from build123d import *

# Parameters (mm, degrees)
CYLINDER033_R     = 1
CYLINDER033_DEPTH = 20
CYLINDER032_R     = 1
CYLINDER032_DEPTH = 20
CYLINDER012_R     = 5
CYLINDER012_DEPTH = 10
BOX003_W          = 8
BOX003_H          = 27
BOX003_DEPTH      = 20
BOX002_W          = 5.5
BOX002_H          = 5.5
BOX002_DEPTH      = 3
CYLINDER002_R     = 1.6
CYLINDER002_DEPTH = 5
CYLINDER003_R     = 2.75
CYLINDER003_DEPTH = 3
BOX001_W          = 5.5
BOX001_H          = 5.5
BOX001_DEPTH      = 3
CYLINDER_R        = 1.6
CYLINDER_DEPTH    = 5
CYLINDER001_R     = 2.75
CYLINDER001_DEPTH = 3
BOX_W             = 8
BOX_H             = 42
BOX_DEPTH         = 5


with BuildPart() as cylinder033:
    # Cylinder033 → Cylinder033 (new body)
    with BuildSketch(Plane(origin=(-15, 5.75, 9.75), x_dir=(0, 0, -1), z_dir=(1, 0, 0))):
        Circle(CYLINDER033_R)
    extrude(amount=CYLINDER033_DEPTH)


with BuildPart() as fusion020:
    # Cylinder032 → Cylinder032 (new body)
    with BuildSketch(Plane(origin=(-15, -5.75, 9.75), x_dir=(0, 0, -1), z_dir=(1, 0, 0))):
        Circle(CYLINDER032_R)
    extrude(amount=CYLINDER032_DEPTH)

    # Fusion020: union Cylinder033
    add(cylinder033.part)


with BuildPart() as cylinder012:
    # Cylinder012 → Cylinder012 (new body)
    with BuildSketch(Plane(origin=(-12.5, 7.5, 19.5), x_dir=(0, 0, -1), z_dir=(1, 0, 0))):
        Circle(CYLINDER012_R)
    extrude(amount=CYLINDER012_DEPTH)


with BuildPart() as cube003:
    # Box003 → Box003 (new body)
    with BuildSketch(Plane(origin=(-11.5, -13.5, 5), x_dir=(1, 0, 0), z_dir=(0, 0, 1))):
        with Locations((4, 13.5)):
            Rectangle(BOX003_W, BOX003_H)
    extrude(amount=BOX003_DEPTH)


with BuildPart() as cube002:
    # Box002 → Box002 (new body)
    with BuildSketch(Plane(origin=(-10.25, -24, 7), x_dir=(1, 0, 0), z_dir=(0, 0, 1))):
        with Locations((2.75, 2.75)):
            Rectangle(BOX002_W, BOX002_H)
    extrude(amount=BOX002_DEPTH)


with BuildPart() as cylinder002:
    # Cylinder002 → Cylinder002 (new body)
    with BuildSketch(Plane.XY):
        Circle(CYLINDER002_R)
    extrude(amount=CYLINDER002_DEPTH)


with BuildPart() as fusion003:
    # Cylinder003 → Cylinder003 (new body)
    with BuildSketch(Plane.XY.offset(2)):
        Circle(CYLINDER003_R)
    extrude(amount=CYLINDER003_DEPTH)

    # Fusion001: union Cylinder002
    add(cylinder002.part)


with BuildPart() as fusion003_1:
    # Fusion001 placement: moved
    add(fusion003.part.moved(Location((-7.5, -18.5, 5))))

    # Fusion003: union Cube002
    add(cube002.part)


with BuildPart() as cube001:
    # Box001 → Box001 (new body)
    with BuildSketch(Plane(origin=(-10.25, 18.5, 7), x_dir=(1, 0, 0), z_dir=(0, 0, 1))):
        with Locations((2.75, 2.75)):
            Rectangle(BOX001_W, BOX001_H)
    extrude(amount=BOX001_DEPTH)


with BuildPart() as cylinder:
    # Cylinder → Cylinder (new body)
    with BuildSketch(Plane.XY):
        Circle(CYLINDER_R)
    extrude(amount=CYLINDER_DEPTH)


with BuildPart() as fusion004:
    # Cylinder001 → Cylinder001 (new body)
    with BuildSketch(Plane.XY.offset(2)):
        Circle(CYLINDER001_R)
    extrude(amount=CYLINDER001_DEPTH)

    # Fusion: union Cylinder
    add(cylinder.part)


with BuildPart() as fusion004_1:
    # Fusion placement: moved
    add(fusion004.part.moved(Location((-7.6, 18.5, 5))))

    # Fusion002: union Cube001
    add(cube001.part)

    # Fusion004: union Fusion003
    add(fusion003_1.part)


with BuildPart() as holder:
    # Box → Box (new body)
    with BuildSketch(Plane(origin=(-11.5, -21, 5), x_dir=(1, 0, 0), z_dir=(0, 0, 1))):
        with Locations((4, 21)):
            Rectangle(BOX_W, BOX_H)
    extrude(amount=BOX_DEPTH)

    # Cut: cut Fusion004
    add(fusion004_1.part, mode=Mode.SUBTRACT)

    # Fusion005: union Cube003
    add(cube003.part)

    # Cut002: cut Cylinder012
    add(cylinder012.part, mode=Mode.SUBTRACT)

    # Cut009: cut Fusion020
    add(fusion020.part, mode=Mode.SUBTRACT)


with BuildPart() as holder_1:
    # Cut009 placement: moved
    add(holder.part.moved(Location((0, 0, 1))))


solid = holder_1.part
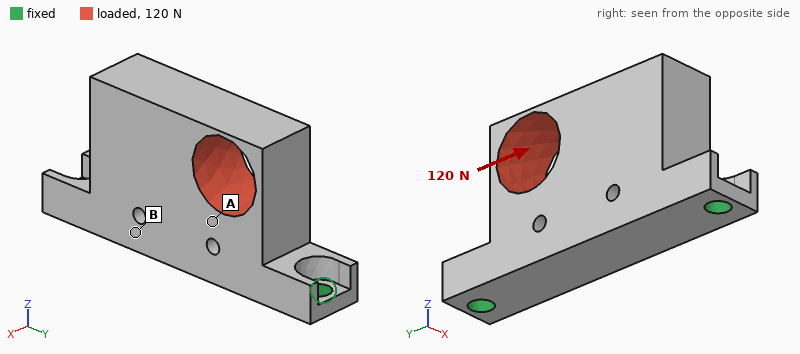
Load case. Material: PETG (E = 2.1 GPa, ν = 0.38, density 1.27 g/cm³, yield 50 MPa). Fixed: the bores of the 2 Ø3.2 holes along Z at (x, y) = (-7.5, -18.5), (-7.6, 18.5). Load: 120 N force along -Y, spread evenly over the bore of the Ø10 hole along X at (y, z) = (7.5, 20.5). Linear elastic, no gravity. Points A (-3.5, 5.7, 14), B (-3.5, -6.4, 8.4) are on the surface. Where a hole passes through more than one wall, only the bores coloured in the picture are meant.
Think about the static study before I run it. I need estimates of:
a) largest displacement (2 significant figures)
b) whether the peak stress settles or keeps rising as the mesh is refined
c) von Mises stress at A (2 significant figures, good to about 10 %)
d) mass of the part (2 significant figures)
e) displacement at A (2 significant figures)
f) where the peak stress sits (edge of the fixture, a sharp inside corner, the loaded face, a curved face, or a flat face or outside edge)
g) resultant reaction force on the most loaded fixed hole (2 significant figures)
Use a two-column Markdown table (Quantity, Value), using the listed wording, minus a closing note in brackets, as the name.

| Quantity | Value |
|---|---|
| largest displacement | 90 µm |
| whether the peak stress settles or keeps rising as the mesh is refined | keeps rising |
| von Mises stress at A | 2.6 MPa |
| mass of the part | 5.2 g |
| displacement at A | 20 µm |
| where the peak stress sits | edge of the fixture |
| resultant reaction force on the most loaded fixed hole | 79 N |
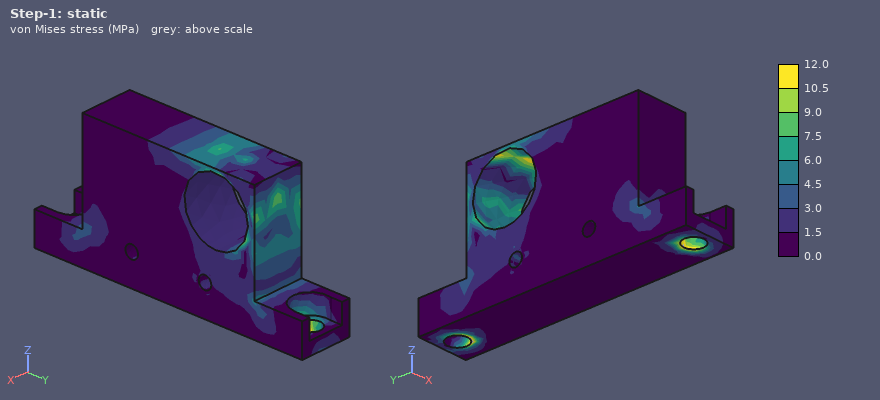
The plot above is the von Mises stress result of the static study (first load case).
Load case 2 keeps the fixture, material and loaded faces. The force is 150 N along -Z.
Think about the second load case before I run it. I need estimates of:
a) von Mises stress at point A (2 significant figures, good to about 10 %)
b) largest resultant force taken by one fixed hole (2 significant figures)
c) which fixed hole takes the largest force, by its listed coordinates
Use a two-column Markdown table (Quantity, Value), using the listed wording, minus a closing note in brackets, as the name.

| Quantity | Value |
|---|---|
| von Mises stress at point A | 2.3 MPa |
| largest resultant force taken by one fixed hole | 130 N |
| which fixed hole takes the largest force, by its listed coordinates | (-7.6, 18.5) |
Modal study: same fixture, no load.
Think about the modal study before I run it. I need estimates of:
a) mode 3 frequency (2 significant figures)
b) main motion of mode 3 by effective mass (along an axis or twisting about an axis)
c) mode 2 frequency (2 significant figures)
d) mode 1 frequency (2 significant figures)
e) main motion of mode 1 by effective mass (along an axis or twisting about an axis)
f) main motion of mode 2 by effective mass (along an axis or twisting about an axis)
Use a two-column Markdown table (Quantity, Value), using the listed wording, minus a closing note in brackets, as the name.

| Quantity | Value |
|---|---|
| mode 3 frequency | 4600 Hz |
| main motion of mode 3 by effective mass | along X |
| mode 2 frequency | 3900 Hz |
| mode 1 frequency | 1100 Hz |
| main motion of mode 1 by effective mass | along X |
| main motion of mode 2 by effective mass | along Z |
